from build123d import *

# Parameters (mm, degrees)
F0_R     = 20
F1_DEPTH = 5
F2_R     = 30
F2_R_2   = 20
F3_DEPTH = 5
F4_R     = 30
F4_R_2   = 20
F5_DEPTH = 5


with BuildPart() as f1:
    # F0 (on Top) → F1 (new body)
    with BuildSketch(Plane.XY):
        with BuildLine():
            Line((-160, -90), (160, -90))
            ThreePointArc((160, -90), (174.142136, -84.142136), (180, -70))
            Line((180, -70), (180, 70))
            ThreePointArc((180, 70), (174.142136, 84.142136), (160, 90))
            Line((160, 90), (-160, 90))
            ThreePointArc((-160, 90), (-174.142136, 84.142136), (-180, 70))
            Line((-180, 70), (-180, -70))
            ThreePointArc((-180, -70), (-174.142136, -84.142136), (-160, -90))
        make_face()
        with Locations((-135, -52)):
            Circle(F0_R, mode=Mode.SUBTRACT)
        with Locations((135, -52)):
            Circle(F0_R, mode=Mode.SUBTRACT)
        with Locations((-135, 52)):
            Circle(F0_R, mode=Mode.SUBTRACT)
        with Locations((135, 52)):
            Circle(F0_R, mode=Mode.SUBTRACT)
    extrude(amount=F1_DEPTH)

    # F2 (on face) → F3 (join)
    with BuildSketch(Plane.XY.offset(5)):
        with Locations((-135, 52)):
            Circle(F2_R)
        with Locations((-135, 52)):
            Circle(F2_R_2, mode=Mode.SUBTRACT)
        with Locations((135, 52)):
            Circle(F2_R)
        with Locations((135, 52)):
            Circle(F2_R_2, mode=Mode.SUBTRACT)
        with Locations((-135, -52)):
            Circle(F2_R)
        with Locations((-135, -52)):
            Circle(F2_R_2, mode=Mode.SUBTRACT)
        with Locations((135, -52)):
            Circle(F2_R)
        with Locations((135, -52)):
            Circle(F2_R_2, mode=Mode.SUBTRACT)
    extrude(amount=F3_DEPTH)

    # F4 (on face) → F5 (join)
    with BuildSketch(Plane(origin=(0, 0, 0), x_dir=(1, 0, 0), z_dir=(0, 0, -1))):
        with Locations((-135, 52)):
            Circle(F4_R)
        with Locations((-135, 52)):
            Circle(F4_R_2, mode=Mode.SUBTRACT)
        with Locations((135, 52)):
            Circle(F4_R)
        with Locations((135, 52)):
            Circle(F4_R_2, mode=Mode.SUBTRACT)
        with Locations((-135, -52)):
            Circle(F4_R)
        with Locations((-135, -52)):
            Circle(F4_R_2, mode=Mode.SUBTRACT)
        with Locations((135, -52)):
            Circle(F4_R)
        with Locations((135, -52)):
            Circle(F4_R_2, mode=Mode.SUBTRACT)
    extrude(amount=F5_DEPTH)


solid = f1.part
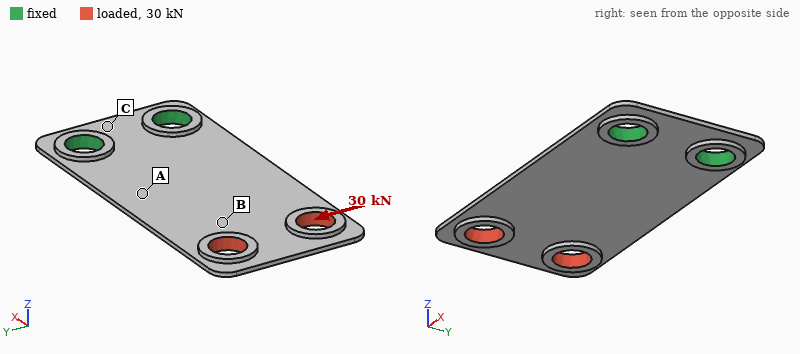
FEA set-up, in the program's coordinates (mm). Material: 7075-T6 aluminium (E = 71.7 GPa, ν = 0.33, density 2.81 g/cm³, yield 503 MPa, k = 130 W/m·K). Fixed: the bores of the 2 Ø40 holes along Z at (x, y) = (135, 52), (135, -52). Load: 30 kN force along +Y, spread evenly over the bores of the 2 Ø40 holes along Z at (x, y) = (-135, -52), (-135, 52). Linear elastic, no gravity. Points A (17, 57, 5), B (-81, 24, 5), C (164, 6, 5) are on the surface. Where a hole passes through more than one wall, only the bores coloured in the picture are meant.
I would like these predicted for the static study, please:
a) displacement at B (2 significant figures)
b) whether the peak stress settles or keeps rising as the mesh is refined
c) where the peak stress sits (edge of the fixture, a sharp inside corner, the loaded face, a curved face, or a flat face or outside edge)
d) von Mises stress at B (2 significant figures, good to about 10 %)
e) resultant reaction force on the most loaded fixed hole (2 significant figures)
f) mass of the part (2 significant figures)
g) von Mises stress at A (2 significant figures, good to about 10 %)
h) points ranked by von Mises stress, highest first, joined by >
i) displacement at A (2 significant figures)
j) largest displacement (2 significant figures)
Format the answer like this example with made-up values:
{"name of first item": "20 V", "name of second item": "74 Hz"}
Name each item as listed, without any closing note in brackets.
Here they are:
{"displacement at B": "0.96 mm", "whether the peak stress settles or keeps rising as the mesh is refined": "keeps rising", "where the peak stress sits": "a sharp inside corner", "von Mises stress at B": "81 MPa", "resultant reaction force on the most loaded fixed hole": "63 kN", "mass of the part": "1.0 kg", "von Mises stress at A": "120 MPa", "points ranked by von Mises stress, highest first, joined by >": "A > B > C", "displacement at A": "0.41 mm", "largest displacement": "1.7 mm"}
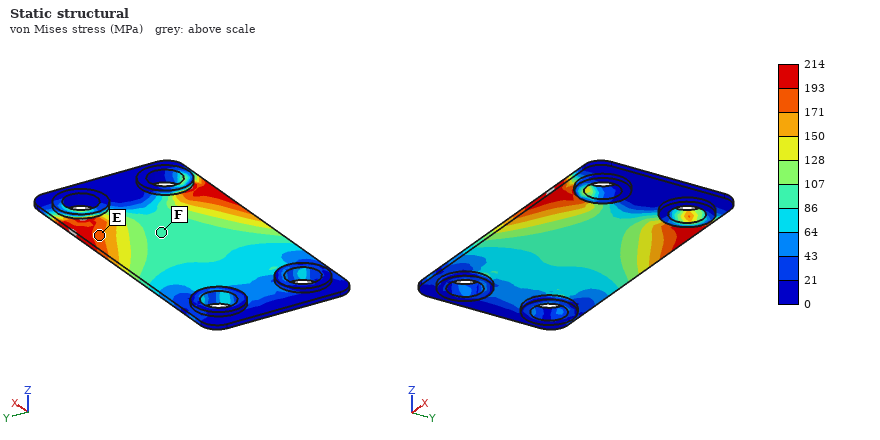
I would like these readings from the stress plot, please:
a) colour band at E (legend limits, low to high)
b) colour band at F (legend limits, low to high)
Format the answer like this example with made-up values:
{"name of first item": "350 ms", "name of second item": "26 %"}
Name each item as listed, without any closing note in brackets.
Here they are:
{"colour band at E": "171 to 193 MPa", "colour band at F": "86 to 107 MPa"}
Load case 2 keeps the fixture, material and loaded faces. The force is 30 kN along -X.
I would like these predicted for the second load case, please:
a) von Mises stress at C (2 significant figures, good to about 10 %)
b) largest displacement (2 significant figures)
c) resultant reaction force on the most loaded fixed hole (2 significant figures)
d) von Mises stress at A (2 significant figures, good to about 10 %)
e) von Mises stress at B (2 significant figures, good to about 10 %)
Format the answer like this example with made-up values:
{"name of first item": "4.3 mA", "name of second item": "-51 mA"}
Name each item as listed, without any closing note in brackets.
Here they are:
{"von Mises stress at C": "4.2 MPa", "largest displacement": "0.13 mm", "resultant reaction force on the most loaded fixed hole": "15 kN", "von Mises stress at A": "33 MPa", "von Mises stress at B": "32 MPa"}
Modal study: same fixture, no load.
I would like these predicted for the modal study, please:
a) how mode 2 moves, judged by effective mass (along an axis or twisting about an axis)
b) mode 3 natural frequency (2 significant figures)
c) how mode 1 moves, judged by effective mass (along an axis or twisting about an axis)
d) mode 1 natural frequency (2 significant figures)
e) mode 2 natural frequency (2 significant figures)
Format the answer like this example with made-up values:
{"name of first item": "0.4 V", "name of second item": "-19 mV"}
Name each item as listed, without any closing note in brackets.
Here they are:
{"how mode 2 moves, judged by effective mass": "twisting about X", "mode 3 natural frequency": "310 Hz", "how mode 1 moves, judged by effective mass": "along Z", "mode 1 natural frequency": "46 Hz", "mode 2 natural frequency": "170 Hz"}
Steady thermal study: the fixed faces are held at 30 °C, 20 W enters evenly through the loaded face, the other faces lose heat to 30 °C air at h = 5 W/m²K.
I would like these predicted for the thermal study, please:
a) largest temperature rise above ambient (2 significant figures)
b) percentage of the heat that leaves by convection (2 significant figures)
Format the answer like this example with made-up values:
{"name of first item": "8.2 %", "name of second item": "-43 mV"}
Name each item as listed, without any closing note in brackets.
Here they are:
{"largest temperature rise above ambient": "29 K", "percentage of the heat that leaves by convection": "43 %"}
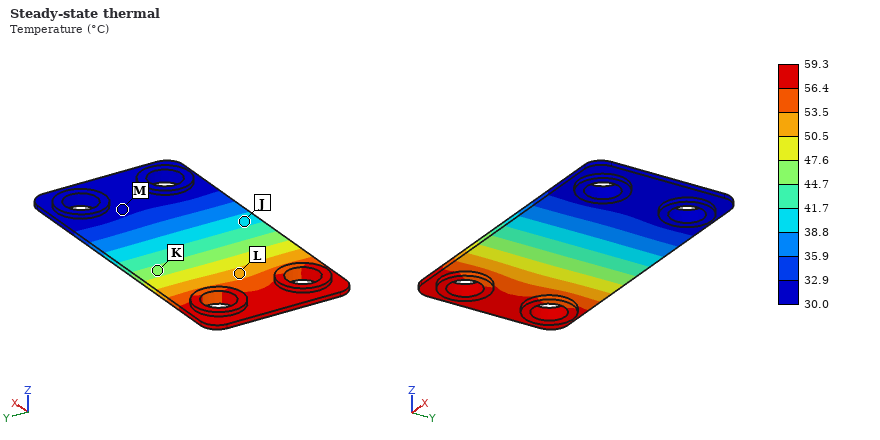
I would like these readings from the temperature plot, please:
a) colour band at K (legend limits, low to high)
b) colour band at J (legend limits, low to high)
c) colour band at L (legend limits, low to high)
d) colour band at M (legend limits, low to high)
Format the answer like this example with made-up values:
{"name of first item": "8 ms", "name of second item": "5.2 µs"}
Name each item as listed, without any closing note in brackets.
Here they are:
{"colour band at K": "44.7 to 47.6 °C", "colour band at J": "38.8 to 41.7 °C", "colour band at L": "50.5 to 53.5 °C", "colour band at M": "30.0 to 32.9 °C"}
